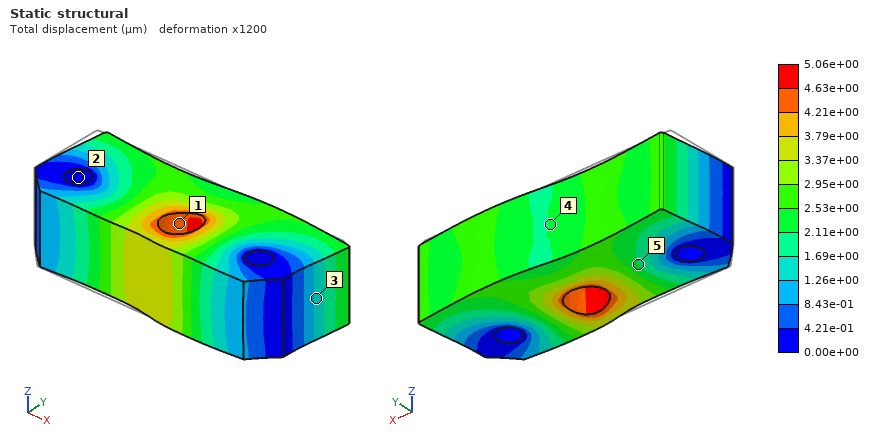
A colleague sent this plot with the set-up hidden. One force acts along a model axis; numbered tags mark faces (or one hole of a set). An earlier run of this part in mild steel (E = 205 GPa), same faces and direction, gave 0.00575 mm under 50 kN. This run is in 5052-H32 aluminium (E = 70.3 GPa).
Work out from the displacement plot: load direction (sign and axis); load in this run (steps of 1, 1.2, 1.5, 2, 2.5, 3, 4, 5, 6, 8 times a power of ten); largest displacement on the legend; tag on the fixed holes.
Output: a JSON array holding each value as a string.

["+X", "15 kN", "5.06e+00 µm", "2"]
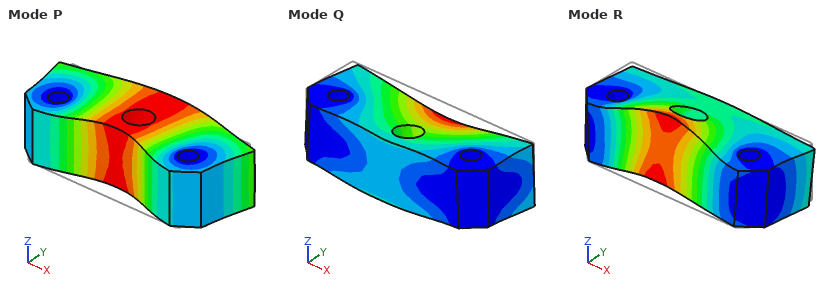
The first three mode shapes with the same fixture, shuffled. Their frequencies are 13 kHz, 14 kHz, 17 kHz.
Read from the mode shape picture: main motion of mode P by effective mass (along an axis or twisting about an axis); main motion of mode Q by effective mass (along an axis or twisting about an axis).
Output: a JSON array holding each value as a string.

["along Y", "along Z"]
